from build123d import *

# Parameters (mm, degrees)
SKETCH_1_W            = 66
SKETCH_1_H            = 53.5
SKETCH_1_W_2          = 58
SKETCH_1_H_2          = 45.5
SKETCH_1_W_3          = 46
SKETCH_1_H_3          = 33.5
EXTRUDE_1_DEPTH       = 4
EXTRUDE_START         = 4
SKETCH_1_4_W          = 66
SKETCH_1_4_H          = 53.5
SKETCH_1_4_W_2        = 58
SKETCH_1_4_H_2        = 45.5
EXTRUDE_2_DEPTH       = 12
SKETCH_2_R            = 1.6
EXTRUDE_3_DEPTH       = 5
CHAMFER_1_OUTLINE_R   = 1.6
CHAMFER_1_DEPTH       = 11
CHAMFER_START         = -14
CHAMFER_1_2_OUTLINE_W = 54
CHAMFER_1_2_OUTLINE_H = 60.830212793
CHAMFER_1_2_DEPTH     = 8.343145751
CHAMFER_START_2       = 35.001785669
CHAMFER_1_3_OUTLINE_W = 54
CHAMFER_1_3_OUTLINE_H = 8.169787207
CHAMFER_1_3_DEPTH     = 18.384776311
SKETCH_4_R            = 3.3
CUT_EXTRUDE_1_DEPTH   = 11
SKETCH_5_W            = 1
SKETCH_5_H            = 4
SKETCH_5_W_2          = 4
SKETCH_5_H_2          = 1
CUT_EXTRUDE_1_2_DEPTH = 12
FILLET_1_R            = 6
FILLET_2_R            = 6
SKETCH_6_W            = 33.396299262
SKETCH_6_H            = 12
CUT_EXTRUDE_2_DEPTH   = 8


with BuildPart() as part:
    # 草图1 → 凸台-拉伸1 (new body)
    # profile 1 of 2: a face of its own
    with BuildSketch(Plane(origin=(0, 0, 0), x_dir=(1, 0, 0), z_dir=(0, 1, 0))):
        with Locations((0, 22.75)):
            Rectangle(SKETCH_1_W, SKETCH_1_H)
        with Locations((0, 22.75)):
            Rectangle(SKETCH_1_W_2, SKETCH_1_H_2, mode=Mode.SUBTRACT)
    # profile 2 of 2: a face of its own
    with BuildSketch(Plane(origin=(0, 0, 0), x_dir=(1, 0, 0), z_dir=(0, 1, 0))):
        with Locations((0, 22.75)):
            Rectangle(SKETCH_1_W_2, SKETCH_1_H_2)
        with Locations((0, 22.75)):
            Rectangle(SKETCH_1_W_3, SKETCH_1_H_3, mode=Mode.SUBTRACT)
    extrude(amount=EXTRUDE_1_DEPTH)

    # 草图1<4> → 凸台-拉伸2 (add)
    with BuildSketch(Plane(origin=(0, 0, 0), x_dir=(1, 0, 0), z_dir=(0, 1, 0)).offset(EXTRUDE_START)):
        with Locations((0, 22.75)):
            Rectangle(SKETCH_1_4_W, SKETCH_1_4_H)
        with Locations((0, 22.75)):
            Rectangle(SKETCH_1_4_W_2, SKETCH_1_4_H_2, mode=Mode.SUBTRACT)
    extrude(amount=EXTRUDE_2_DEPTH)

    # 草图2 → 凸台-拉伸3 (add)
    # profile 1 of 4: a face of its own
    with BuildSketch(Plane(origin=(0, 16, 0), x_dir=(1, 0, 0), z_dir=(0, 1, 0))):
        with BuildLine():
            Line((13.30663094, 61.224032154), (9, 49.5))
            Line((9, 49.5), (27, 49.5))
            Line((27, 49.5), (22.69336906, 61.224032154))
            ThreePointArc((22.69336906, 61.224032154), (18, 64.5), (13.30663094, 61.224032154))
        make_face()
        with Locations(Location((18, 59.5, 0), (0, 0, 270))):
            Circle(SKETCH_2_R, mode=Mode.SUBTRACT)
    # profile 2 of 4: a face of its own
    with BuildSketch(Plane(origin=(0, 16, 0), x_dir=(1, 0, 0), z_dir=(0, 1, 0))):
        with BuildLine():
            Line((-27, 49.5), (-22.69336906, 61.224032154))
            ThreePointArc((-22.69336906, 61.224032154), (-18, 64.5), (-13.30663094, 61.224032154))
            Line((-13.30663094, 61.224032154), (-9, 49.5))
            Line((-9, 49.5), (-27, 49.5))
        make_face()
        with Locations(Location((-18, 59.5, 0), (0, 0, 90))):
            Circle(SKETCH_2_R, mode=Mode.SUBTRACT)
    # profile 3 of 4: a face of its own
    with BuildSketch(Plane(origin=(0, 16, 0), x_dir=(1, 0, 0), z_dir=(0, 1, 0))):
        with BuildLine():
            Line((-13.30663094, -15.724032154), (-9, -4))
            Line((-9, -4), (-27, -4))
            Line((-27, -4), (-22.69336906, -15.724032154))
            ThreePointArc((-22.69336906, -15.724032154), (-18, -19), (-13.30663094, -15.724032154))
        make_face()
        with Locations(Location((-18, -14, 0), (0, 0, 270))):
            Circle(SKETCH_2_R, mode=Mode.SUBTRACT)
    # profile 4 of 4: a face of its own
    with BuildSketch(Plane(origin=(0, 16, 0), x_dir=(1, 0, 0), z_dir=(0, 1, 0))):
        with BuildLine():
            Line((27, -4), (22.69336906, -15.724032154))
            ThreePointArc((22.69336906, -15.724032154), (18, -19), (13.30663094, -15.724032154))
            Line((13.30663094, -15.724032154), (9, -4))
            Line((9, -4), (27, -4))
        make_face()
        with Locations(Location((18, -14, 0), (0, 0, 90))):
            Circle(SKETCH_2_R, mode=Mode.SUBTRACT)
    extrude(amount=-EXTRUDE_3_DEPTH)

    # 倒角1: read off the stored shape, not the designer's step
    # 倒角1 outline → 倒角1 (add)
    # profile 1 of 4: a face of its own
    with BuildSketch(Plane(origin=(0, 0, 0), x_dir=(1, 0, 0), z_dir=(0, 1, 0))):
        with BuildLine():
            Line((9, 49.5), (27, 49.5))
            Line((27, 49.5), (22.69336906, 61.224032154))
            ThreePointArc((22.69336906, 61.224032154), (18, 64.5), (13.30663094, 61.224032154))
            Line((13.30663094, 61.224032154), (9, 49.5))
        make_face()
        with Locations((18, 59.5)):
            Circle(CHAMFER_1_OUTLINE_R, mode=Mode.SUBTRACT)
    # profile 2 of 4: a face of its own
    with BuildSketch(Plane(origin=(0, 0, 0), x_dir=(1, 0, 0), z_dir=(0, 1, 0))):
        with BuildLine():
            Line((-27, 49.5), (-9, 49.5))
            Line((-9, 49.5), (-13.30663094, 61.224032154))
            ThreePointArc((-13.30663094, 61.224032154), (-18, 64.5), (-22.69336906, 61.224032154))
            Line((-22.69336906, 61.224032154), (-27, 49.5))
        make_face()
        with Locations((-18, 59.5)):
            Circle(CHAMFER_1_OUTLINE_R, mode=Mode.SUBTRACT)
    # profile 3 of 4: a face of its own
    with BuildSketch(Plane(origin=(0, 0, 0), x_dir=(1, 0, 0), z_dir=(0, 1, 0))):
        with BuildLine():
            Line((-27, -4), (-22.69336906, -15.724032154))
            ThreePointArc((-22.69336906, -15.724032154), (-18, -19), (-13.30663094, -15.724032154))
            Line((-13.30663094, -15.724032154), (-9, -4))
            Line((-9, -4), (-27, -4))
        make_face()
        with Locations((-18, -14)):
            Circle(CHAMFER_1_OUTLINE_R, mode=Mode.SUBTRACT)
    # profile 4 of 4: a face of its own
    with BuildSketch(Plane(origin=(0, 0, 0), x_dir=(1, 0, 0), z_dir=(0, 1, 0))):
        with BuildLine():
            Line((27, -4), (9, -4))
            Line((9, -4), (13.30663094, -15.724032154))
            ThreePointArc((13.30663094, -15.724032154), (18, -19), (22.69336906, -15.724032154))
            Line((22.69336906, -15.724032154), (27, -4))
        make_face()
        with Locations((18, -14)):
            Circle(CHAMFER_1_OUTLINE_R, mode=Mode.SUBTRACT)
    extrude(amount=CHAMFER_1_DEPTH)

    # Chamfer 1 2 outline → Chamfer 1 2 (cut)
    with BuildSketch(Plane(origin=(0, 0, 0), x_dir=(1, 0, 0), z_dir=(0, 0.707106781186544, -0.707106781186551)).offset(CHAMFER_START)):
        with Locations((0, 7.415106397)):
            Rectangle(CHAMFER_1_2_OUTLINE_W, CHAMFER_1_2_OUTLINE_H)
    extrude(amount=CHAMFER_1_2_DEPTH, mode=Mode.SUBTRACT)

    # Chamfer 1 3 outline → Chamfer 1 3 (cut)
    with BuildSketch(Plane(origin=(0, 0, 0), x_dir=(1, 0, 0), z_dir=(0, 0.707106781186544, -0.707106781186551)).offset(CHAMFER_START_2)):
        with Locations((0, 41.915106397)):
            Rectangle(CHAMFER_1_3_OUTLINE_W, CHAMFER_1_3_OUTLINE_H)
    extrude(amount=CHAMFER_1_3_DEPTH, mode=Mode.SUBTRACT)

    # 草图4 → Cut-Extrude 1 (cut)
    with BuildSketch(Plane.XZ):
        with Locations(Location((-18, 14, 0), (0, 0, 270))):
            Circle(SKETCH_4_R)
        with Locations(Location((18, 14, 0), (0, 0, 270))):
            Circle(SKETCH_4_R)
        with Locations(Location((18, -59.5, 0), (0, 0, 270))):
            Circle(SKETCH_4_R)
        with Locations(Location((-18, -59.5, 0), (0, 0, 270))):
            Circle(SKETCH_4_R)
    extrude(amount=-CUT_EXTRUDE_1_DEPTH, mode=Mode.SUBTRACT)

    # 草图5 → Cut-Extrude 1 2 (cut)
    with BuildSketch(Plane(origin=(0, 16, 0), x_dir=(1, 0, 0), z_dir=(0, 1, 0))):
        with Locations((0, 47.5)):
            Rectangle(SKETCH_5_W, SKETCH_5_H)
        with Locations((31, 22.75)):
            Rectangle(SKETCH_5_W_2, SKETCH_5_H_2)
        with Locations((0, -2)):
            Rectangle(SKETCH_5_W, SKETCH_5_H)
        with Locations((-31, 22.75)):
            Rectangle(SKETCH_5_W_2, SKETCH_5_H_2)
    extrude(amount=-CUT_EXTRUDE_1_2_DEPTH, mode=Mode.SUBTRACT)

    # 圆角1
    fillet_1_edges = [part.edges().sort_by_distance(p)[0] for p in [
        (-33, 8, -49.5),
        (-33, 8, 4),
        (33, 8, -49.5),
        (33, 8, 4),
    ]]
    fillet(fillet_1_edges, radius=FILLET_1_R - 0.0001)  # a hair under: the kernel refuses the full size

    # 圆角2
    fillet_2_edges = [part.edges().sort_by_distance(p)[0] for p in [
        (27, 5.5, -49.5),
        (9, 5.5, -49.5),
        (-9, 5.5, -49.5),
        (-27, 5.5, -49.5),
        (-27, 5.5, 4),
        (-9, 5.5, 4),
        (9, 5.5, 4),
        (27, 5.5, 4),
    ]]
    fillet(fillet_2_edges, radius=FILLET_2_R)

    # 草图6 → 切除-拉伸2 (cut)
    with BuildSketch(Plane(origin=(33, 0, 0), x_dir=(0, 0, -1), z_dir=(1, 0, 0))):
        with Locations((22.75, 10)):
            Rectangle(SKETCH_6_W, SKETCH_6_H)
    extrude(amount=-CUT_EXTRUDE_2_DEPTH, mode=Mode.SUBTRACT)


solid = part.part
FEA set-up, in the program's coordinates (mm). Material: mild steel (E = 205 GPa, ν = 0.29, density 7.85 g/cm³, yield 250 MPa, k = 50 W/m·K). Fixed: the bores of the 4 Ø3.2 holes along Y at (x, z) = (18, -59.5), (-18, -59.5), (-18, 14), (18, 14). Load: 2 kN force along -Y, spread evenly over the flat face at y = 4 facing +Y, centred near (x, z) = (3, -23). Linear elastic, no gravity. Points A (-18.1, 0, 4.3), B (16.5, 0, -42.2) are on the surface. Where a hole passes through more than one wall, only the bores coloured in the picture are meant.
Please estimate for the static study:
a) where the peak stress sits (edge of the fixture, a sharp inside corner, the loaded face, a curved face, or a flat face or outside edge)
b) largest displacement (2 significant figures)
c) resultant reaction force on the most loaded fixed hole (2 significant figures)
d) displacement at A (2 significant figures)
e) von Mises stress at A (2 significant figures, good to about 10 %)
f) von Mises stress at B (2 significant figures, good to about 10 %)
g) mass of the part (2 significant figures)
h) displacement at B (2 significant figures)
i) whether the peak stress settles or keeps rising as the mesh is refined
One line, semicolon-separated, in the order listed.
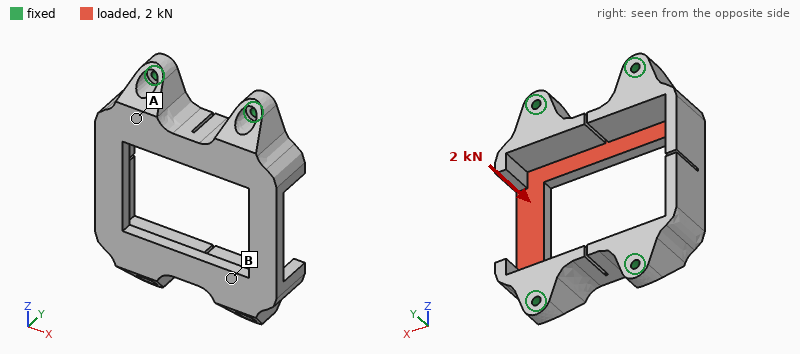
edge of the fixture; 23 µm; 910 N; 5.0 µm; 6.7 MPa; 12 MPa; 200 g; 9.2 µm; keeps rising
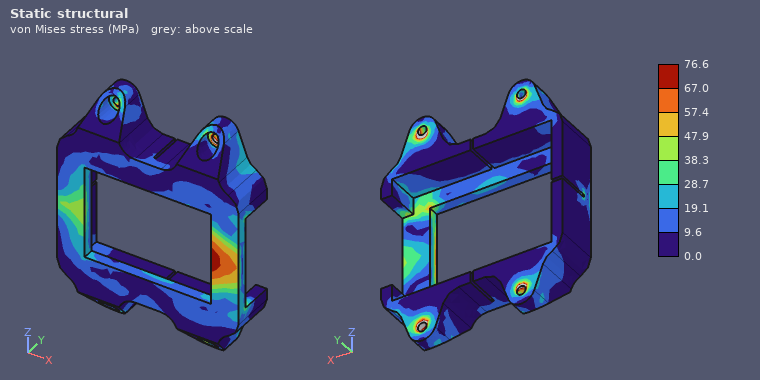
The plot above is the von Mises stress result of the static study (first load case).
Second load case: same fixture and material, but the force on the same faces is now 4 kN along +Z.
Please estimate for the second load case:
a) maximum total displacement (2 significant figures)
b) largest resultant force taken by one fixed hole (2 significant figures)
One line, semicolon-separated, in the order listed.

20 µm; 1.0 kN
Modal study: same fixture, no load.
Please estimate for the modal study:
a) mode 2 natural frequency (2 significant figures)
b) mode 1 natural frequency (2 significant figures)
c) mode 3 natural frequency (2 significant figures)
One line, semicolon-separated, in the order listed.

6900 Hz; 6400 Hz; 7400 Hz
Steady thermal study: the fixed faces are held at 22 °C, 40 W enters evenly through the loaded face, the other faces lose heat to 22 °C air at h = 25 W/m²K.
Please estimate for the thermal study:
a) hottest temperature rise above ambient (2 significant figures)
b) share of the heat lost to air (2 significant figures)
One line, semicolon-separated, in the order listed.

61 K; 15 %
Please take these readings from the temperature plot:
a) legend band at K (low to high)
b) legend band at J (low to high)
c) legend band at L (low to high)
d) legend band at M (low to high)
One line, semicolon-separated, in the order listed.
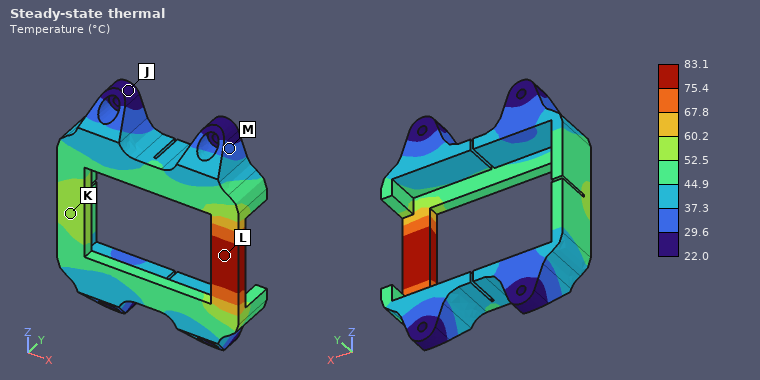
52.5 to 60.2 °C; 22.0 to 29.6 °C; 75.4 to 83.1 °C; 29.6 to 37.3 °C
